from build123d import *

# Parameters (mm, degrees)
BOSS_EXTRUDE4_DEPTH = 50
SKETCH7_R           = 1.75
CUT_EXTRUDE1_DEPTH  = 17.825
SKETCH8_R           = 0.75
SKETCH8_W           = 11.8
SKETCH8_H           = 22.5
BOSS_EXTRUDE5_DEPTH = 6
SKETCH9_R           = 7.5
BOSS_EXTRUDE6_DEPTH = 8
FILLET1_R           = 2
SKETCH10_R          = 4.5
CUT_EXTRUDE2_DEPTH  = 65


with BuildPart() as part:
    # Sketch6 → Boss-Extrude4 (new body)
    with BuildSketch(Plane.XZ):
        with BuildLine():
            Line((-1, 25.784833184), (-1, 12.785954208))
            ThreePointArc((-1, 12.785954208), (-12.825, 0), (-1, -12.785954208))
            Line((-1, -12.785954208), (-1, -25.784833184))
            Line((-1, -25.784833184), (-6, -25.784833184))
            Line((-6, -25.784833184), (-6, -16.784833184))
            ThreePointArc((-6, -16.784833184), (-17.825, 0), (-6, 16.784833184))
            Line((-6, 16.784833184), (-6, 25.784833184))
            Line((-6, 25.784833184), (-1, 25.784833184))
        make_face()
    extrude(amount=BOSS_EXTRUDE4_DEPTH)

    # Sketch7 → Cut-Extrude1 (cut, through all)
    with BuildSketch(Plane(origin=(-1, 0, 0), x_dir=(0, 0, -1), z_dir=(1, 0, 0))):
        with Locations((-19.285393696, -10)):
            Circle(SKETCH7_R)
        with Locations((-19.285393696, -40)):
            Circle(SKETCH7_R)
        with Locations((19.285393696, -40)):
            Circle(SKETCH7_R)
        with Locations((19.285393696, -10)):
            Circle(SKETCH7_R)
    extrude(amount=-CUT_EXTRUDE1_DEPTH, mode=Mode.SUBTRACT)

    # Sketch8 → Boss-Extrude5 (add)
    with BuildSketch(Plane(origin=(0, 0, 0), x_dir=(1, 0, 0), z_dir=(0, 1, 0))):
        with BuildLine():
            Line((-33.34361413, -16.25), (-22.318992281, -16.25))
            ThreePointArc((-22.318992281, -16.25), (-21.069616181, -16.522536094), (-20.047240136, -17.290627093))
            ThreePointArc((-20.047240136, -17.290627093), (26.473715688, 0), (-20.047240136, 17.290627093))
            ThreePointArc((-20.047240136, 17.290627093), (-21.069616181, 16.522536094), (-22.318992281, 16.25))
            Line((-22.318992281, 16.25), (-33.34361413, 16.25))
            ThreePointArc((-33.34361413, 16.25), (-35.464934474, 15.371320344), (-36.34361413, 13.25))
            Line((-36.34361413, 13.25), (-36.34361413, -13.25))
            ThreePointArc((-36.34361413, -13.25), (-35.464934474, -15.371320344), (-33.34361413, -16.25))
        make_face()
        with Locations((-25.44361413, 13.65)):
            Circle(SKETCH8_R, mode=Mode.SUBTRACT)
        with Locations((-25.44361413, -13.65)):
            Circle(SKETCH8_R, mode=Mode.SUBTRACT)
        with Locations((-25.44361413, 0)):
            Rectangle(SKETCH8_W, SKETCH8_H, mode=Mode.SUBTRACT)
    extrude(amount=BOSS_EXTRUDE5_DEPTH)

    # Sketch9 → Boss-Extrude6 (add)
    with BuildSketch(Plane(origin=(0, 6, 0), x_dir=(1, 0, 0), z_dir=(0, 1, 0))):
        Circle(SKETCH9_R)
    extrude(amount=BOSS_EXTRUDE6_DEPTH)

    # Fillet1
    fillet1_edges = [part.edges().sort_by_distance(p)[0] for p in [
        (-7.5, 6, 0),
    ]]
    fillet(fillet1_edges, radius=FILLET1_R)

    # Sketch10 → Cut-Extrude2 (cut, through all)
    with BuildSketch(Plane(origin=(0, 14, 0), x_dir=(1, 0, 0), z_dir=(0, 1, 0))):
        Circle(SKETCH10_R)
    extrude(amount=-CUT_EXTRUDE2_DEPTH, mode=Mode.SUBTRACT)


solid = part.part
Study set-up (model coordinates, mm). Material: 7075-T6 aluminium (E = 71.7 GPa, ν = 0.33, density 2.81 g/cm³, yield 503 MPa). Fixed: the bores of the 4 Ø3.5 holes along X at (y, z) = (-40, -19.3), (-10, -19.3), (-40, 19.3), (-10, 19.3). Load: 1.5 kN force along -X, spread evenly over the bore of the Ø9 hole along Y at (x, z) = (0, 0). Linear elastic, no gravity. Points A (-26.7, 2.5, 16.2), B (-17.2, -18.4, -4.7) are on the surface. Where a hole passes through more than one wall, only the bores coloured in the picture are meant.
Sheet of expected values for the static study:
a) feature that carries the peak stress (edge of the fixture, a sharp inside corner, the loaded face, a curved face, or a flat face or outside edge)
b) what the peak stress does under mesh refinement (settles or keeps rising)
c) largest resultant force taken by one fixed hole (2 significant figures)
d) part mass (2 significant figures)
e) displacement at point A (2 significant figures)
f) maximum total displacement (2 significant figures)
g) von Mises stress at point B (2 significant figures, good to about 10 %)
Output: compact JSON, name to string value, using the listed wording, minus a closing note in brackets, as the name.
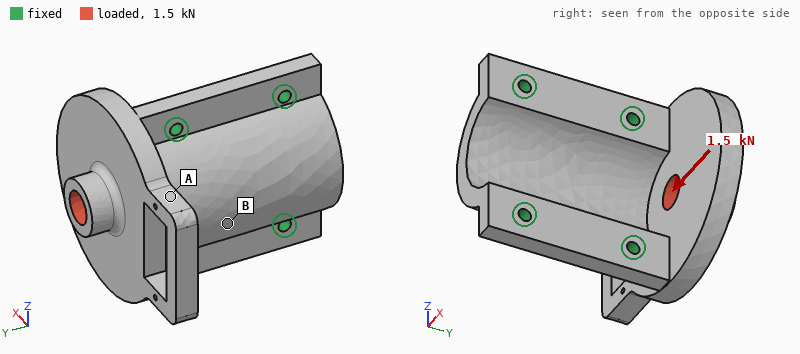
{"feature that carries the peak stress": "edge of the fixture", "what the peak stress does under mesh refinement": "keeps rising", "largest resultant force taken by one fixed hole": "1.4 kN", "part mass": "84 g", "displacement at point A": "32 µm", "maximum total displacement": "67 µm", "von Mises stress at point B": "17 MPa"}
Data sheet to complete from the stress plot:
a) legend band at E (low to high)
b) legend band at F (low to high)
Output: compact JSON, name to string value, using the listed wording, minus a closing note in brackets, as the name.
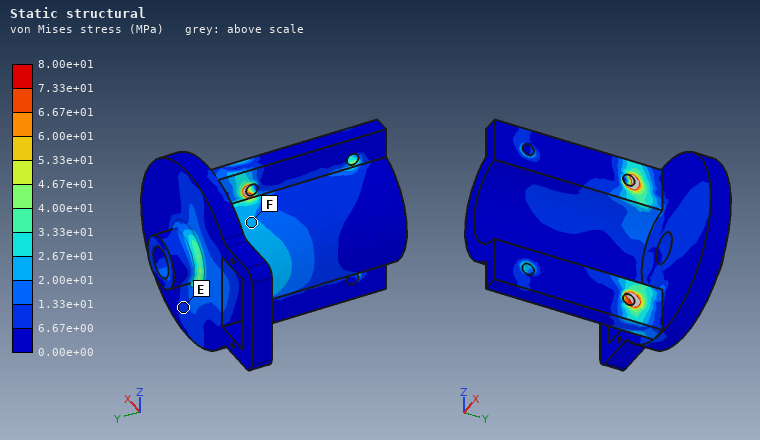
{"legend band at E": "6.67e+00 to 1.33e+01 MPa", "legend band at F": "2.00e+01 to 2.67e+01 MPa"}
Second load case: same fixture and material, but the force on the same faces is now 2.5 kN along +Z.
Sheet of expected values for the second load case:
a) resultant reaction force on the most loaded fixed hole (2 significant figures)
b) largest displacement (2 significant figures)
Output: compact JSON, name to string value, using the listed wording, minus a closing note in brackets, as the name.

{"resultant reaction force on the most loaded fixed hole": "1.5 kN", "largest displacement": "30 µm"}
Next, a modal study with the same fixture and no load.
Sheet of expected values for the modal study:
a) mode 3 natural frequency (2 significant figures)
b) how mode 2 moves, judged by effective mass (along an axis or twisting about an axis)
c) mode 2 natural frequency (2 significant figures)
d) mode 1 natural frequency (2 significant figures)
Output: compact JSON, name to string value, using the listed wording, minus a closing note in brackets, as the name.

{"mode 3 natural frequency": "6900 Hz", "how mode 2 moves, judged by effective mass": "along Y", "mode 2 natural frequency": "6200 Hz", "mode 1 natural frequency": "4100 Hz"}
